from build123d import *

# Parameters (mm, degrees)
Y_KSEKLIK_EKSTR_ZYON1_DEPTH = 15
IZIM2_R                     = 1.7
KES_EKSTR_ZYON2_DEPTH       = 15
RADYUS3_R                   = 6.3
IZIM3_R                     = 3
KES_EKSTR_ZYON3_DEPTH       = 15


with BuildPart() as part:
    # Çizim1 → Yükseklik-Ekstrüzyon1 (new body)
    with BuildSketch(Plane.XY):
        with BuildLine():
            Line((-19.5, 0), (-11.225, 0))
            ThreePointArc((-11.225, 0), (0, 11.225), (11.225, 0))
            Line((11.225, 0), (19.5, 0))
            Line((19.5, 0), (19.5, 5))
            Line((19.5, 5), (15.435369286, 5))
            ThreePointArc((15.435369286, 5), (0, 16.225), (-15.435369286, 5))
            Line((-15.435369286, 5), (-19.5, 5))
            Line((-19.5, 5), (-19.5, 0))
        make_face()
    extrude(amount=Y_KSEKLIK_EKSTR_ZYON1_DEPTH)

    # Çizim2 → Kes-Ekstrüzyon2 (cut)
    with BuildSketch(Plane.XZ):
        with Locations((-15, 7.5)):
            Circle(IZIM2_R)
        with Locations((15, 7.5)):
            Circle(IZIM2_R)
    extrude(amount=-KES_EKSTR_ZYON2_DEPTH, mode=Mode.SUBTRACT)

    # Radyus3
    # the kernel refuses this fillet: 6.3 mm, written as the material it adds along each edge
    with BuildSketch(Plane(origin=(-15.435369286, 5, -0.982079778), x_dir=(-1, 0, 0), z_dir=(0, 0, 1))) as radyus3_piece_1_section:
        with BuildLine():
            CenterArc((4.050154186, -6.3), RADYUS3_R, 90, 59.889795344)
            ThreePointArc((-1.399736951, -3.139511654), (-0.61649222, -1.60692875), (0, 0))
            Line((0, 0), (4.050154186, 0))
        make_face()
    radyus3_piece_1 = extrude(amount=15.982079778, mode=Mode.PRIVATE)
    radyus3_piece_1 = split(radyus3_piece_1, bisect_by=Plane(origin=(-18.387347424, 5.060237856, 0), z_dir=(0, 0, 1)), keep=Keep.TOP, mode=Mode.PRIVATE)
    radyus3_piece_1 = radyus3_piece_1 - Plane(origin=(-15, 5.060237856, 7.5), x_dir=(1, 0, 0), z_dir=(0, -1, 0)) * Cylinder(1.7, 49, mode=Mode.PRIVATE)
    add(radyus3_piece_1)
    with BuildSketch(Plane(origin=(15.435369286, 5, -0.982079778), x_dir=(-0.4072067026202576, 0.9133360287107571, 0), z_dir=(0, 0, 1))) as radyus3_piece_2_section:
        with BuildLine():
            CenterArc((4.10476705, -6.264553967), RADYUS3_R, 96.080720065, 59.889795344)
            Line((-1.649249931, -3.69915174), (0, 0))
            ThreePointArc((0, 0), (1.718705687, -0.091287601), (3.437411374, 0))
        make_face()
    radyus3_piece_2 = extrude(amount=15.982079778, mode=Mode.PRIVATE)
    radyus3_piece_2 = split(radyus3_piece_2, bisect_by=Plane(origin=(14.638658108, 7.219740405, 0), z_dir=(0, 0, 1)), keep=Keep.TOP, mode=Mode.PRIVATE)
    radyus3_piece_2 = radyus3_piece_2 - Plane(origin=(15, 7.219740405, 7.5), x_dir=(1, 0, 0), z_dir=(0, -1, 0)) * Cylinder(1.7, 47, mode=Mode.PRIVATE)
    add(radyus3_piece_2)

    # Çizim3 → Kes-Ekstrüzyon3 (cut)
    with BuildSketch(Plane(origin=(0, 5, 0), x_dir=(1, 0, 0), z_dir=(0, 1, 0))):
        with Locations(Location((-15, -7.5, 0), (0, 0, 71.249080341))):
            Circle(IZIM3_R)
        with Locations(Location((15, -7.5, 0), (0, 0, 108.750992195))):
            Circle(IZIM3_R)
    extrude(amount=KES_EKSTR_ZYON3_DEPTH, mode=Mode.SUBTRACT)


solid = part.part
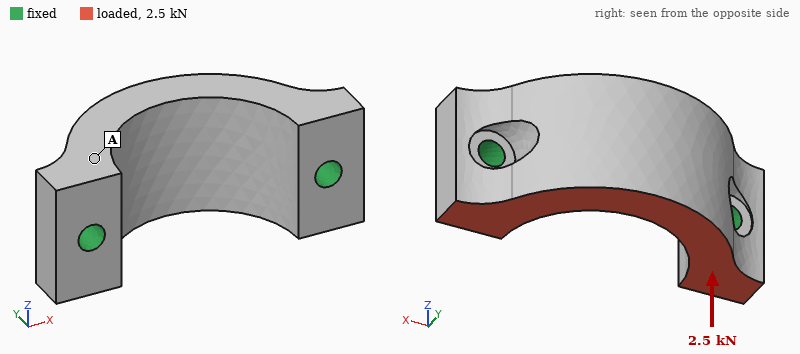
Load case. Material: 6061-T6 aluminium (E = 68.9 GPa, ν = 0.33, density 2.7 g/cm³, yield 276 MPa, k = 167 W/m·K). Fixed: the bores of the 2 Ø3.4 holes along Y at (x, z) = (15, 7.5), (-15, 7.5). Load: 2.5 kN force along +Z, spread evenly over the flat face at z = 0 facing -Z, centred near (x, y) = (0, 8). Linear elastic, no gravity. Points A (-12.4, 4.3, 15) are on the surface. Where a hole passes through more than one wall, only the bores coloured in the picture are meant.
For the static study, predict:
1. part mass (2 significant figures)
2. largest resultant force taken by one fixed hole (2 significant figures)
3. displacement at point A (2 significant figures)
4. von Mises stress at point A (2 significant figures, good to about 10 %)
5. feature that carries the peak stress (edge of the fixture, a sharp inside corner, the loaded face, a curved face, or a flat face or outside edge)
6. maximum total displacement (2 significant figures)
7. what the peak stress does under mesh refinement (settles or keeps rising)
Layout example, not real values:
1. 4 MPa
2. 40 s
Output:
1. 9.8 g
2. 1.3 kN
3. 14 µm
4. 28 MPa
5. edge of the fixture
6. 41 µm
7. keeps rising
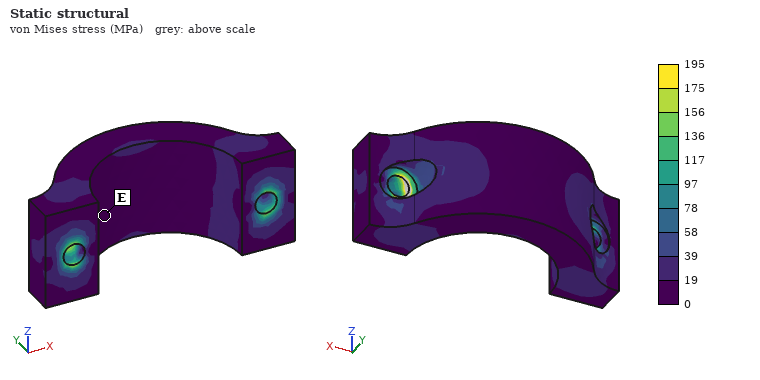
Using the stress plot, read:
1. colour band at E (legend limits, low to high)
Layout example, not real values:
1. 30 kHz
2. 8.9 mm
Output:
1. 0 to 19 MPa
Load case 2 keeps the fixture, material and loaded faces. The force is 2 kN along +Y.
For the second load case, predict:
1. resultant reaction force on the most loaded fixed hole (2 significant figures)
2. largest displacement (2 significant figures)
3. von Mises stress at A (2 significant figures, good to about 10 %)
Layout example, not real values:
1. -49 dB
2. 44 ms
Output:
1. 1.1 kN
2. 40 µm
3. 25 MPa
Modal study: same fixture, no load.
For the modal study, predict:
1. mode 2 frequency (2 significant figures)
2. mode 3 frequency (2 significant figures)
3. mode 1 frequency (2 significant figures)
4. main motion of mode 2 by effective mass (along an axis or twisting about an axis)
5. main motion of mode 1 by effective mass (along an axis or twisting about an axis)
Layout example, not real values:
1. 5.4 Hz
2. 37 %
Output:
1. 26 kHz
2. 32 kHz
3. 15 kHz
4. along X
5. along Z
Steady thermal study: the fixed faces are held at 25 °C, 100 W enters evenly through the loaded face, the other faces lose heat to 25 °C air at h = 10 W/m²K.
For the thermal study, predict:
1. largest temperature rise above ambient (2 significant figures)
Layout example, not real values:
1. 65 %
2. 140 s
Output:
1. 49 K
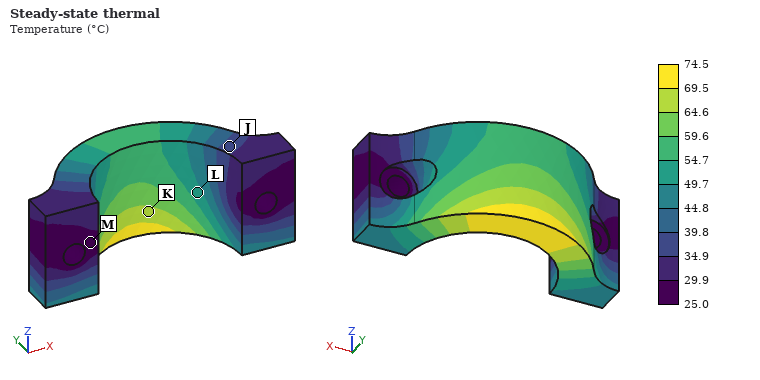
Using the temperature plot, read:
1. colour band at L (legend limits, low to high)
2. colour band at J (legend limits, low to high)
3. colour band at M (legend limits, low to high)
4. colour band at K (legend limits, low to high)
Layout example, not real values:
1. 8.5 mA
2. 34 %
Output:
1. 49.7 to 54.7 °C
2. 34.9 to 39.8 °C
3. 25.0 to 29.9 °C
4. 64.6 to 69.5 °C
